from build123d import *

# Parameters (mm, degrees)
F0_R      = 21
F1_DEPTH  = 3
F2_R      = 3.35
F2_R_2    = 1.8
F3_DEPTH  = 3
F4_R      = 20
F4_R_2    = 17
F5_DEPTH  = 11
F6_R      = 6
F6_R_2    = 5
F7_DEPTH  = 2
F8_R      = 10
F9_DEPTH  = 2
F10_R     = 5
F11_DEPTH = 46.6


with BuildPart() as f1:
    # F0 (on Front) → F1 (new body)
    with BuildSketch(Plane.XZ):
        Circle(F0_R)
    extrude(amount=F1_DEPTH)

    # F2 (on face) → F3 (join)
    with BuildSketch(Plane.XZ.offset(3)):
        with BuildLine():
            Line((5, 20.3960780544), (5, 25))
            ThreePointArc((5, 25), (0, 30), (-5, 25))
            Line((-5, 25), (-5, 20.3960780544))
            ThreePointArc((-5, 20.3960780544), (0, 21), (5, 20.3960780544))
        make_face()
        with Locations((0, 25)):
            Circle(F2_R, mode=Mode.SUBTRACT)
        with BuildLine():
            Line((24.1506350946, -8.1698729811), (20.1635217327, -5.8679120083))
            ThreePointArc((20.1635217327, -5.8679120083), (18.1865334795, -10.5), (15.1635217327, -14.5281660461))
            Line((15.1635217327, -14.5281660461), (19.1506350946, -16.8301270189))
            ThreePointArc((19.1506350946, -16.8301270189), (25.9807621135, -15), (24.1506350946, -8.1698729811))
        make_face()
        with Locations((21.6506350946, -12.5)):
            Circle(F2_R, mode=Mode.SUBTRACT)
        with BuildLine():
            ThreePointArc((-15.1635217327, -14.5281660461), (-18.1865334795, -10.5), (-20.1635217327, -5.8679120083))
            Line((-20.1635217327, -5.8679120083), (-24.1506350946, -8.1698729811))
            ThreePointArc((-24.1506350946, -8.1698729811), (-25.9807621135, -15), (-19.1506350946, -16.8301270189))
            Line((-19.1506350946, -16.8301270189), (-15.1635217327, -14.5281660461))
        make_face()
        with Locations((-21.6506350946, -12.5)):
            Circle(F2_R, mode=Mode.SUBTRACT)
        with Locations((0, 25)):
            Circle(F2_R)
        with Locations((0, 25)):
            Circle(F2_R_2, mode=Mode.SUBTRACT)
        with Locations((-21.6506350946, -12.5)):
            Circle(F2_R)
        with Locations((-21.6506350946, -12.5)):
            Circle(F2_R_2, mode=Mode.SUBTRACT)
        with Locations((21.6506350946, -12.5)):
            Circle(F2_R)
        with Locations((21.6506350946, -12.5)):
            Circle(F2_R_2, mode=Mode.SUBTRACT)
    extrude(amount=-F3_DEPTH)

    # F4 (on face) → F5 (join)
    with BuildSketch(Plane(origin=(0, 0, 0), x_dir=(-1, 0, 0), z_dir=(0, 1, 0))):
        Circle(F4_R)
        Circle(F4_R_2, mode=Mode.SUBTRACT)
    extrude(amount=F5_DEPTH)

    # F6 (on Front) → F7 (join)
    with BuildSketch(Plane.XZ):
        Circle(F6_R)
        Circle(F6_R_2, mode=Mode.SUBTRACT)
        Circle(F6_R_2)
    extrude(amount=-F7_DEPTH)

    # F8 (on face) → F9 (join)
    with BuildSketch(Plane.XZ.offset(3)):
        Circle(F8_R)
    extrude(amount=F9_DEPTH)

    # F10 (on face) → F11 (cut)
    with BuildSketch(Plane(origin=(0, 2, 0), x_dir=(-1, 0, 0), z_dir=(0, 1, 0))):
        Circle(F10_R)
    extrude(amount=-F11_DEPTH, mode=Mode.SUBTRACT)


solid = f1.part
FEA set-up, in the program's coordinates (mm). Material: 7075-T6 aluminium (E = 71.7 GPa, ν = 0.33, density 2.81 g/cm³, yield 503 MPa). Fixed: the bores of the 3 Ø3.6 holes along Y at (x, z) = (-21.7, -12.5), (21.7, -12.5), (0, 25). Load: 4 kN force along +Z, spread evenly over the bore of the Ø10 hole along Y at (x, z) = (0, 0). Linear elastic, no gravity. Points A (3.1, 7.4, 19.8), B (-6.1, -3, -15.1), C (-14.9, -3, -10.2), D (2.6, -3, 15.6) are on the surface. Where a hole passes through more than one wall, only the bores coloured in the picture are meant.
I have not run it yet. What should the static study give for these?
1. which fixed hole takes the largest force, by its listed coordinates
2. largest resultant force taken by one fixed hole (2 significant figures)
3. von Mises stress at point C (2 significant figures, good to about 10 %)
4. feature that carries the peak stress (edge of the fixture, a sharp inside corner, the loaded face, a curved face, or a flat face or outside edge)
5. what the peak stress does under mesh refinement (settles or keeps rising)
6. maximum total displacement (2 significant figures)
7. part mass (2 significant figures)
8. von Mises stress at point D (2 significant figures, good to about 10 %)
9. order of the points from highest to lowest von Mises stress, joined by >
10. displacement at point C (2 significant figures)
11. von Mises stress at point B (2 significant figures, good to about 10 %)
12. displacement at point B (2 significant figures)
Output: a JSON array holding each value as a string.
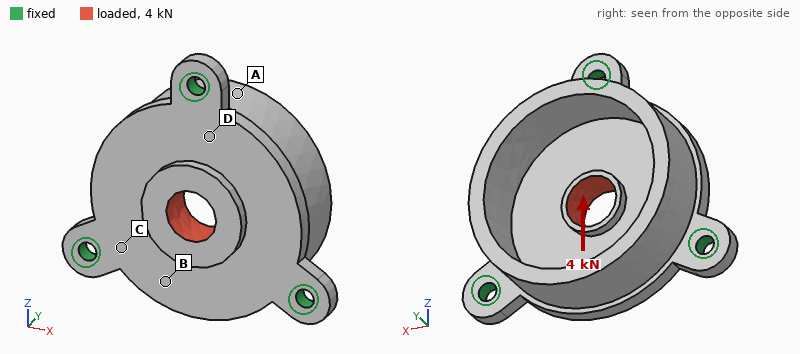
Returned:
["(0, 25)", "1.8 kN", "31 MPa", "edge of the fixture", "keeps rising", "30 µm", "25 g", "52 MPa", "D > C > B > A", "8.7 µm", "19 MPa", "16 µm"]
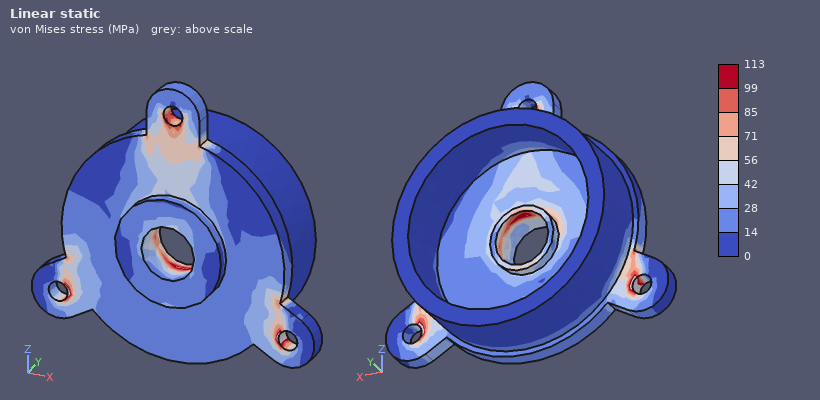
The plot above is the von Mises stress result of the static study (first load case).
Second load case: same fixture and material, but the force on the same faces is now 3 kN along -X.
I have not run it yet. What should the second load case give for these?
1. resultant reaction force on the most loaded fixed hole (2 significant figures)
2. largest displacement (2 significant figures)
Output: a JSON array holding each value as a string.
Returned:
["1.2 kN", "20 µm"]
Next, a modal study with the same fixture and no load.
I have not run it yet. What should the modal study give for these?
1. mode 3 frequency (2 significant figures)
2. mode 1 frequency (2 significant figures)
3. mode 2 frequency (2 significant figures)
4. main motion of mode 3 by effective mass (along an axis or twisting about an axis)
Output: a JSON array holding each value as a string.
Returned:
["9800 Hz", "8100 Hz", "8100 Hz", "along Y"]
